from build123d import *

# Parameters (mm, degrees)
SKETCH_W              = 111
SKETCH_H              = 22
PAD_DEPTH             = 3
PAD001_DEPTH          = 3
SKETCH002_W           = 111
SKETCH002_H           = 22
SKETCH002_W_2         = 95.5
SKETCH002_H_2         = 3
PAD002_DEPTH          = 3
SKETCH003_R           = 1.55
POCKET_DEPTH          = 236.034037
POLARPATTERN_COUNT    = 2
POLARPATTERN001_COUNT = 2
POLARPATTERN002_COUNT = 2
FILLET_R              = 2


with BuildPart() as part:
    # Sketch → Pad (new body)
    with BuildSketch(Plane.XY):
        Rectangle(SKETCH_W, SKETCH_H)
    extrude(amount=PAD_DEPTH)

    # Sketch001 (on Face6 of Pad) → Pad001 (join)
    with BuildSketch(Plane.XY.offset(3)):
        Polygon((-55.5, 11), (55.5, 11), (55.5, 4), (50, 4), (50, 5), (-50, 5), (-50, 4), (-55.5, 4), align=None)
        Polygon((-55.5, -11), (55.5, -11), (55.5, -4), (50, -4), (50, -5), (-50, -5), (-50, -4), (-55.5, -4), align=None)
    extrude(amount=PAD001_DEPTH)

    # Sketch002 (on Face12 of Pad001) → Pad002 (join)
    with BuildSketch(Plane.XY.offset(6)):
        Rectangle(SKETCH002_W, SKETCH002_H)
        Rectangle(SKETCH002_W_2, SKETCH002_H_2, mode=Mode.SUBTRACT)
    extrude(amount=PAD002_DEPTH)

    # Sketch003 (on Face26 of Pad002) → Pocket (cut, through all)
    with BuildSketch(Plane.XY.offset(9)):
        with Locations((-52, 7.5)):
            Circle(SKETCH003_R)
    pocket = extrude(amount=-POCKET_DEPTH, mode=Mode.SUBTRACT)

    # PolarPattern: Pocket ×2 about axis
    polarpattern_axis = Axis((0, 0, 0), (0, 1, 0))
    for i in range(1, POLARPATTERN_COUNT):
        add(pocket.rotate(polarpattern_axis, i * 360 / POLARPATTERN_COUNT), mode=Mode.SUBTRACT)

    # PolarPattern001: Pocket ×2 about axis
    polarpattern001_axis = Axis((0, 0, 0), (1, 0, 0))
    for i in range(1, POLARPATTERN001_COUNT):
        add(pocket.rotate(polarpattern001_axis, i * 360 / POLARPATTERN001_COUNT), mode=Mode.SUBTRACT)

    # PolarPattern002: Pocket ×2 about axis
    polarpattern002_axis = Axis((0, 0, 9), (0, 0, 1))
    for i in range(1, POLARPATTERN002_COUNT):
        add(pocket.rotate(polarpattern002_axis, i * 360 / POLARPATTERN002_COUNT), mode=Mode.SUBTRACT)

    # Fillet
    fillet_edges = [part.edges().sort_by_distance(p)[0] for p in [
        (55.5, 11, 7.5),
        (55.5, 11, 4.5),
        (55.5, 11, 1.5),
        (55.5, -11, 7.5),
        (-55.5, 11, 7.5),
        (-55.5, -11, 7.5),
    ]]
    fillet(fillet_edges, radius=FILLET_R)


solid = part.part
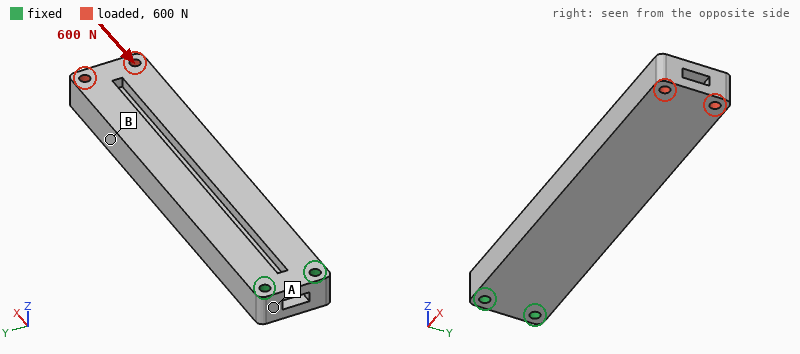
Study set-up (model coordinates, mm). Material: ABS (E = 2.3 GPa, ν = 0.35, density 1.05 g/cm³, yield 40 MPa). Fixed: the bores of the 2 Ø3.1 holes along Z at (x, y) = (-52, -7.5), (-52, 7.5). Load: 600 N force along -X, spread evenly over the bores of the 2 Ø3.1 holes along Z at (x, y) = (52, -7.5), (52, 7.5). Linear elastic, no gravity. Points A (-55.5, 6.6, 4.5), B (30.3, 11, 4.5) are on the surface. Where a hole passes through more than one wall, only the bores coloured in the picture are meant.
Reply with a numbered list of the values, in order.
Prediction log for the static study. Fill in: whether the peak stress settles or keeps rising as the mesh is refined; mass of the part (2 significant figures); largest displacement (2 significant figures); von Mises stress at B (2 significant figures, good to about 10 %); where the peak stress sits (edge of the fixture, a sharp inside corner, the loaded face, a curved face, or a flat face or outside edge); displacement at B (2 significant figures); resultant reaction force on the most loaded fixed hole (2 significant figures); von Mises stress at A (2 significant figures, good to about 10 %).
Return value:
1. keeps rising
2. 18 g
3. 0.27 mm
4. 3.8 MPa
5. edge of the fixture
6. 0.17 mm
7. 300 N
8. 1.5 MPa
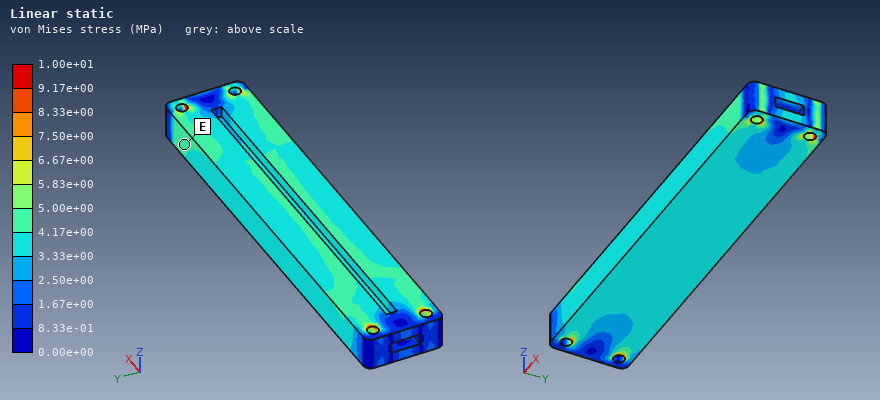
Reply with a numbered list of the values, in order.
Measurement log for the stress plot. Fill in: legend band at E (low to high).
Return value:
1. 4.17e+00 to 5.00e+00 MPa
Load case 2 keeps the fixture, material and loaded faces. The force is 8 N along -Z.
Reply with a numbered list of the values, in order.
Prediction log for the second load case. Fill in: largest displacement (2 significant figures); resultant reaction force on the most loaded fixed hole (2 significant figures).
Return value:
1. 1.2 mm
2. 5.6 N
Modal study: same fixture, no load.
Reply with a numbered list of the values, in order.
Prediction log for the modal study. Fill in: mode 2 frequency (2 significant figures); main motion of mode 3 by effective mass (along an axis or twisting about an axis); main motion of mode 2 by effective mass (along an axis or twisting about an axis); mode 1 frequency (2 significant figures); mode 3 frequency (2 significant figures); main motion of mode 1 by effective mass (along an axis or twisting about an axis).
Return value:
1. 440 Hz
2. twisting about X
3. along Y
4. 200 Hz
5. 930 Hz
6. along Z
